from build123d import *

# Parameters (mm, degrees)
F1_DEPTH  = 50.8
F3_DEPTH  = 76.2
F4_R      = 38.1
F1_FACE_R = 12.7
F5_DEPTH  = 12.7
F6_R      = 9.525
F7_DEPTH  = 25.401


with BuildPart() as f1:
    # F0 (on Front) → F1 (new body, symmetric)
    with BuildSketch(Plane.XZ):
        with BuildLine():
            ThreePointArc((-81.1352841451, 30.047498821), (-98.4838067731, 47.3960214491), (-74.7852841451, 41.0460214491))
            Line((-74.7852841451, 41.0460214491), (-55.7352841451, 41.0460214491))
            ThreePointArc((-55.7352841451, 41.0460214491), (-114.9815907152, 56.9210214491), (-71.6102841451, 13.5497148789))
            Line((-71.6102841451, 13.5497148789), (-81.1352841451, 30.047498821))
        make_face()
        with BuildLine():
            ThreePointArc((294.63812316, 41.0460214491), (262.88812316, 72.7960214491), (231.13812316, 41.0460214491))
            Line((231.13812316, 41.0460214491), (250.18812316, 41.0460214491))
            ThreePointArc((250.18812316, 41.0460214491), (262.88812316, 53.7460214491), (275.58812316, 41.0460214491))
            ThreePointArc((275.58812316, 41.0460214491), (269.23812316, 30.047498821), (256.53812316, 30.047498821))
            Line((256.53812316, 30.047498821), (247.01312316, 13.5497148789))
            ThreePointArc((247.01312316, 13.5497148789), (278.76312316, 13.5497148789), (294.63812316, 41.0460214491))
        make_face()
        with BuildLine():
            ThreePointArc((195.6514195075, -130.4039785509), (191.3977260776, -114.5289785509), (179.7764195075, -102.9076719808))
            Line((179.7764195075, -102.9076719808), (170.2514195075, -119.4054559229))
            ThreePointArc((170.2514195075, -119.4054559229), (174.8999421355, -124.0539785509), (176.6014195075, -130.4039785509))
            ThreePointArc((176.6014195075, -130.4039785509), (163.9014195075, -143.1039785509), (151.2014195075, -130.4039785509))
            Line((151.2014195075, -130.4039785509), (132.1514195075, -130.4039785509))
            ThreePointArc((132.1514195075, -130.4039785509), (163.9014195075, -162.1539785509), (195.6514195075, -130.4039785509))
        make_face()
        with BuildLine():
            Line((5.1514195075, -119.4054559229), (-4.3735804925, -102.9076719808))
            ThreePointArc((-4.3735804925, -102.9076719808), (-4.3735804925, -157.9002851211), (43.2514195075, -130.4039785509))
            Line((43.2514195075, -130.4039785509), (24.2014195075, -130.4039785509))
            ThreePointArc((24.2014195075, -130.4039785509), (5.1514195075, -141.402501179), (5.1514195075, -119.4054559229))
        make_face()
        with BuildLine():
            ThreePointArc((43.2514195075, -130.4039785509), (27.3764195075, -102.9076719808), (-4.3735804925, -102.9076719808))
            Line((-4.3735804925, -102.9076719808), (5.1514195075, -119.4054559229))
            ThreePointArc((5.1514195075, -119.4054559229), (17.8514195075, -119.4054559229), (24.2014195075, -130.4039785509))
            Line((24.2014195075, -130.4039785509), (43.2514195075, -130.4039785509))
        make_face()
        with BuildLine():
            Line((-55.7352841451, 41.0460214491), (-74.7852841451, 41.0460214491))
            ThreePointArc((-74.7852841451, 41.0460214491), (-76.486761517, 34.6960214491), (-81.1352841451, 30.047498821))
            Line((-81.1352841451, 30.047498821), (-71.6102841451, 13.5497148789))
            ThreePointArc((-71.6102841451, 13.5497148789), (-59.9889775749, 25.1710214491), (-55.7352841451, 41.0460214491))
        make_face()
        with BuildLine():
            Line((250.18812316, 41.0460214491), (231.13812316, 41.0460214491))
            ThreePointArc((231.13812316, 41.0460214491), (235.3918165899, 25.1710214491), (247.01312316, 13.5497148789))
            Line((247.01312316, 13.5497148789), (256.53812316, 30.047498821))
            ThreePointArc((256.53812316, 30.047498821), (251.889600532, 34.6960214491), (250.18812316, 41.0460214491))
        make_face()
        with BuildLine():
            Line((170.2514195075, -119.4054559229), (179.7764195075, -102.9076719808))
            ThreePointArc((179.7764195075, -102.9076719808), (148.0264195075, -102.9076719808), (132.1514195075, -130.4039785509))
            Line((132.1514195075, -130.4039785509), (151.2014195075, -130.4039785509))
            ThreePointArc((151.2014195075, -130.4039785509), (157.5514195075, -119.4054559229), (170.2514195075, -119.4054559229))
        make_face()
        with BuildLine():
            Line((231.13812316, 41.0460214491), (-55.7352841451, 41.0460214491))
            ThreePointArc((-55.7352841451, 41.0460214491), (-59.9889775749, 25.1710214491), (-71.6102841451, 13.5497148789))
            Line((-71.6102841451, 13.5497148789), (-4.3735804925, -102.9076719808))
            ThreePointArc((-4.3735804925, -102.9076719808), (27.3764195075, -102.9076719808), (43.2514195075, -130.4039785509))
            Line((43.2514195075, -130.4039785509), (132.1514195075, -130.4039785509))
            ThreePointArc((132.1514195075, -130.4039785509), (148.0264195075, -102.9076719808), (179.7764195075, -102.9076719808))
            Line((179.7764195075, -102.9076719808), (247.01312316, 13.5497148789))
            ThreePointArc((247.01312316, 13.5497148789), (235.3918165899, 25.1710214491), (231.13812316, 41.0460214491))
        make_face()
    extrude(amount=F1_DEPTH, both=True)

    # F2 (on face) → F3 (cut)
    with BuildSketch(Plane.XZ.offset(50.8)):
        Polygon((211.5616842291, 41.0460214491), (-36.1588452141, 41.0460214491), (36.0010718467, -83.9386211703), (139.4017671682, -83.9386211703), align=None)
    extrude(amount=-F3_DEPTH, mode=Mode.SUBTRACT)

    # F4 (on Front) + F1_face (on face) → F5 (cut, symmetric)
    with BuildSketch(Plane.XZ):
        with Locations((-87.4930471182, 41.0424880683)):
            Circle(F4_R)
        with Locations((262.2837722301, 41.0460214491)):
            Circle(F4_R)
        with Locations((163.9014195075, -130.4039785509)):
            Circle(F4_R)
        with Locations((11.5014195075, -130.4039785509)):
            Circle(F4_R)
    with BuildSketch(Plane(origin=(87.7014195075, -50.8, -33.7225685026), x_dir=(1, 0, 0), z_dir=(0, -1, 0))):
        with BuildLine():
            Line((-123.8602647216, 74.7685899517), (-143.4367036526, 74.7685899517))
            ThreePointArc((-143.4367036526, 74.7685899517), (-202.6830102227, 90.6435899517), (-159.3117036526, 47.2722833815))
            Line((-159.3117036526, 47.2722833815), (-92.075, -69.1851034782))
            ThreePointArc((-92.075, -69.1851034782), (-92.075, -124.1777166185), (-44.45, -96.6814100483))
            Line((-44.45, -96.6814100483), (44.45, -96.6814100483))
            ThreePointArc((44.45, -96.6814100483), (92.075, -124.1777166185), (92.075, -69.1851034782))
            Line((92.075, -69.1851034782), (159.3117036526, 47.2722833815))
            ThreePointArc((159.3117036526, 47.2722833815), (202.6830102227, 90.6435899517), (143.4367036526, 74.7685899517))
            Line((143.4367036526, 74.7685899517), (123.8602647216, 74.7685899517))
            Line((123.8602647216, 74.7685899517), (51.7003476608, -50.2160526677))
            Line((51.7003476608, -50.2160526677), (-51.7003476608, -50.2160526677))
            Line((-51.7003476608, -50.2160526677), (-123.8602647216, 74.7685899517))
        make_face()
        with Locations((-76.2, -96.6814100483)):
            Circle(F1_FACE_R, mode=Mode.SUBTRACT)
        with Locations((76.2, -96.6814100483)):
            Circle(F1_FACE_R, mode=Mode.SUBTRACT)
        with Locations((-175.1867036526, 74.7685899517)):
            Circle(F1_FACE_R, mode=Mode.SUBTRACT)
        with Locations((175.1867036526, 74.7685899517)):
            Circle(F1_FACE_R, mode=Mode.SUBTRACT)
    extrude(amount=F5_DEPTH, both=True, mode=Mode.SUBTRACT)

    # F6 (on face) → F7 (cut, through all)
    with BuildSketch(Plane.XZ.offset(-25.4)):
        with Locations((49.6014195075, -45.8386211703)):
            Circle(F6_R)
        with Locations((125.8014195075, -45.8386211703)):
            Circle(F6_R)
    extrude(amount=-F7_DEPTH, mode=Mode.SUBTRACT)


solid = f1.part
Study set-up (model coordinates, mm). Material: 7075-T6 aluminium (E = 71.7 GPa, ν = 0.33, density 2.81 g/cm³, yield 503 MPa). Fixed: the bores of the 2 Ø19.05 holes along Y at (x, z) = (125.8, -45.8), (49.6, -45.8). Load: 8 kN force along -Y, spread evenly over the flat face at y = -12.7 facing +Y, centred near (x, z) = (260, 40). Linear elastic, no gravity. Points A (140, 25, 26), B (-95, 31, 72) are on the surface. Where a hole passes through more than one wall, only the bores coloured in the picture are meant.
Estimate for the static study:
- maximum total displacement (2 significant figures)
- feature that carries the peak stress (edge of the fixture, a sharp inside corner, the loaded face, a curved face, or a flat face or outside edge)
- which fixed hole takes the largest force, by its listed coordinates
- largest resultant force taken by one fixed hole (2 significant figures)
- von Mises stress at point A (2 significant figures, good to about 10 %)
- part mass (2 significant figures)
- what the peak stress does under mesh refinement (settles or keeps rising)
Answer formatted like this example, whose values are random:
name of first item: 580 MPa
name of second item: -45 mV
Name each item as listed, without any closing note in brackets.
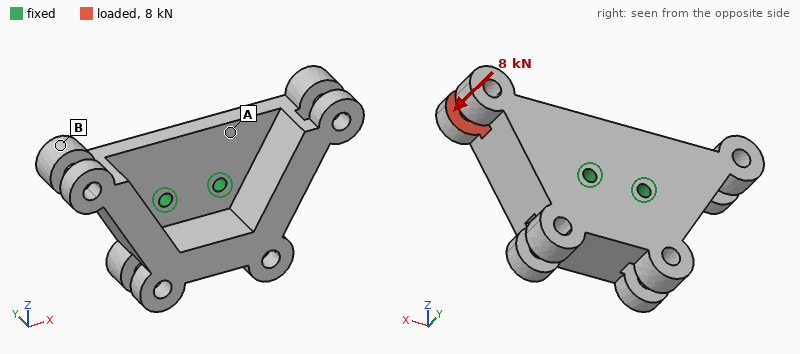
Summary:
maximum total displacement: 0.50 mm
feature that carries the peak stress: edge of the fixture
which fixed hole takes the largest force, by its listed coordinates: (125.8, -45.8)
largest resultant force taken by one fixed hole: 17 kN
von Mises stress at point A: 16 MPa
part mass: 7.8 kg
what the peak stress does under mesh refinement: keeps rising
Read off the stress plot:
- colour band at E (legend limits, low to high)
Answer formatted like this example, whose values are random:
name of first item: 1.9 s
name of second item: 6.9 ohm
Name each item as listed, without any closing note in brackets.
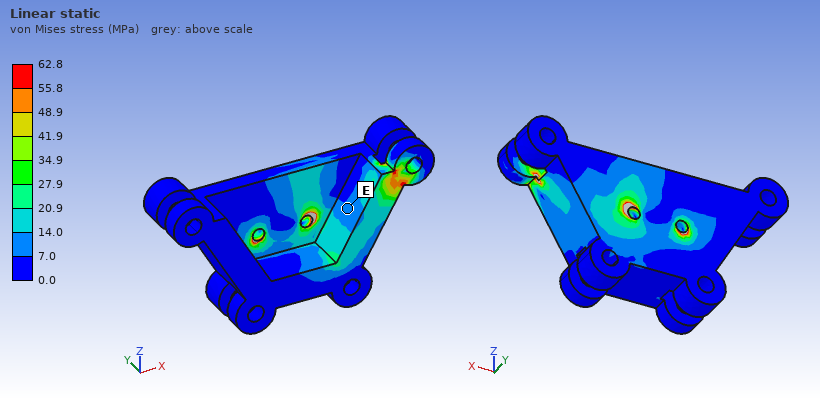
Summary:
colour band at E: 7.0 to 14.0 MPa
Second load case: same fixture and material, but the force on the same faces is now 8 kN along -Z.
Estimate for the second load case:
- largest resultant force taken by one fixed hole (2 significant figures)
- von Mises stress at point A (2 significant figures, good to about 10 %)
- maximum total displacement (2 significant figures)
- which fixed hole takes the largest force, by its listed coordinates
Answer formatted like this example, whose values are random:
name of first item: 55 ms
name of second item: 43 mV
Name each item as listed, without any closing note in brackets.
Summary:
largest resultant force taken by one fixed hole: 19 kN
von Mises stress at point A: 10 MPa
maximum total displacement: 0.26 mm
which fixed hole takes the largest force, by its listed coordinates: (125.8, -45.8)
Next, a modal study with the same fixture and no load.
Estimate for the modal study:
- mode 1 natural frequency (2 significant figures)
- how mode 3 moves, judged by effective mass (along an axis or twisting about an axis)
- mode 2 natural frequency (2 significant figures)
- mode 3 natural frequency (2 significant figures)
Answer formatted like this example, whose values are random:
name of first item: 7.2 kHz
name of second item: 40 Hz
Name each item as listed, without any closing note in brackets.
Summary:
mode 1 natural frequency: 760 Hz
how mode 3 moves, judged by effective mass: twisting about Y
mode 2 natural frequency: 900 Hz
mode 3 natural frequency: 1300 Hz
